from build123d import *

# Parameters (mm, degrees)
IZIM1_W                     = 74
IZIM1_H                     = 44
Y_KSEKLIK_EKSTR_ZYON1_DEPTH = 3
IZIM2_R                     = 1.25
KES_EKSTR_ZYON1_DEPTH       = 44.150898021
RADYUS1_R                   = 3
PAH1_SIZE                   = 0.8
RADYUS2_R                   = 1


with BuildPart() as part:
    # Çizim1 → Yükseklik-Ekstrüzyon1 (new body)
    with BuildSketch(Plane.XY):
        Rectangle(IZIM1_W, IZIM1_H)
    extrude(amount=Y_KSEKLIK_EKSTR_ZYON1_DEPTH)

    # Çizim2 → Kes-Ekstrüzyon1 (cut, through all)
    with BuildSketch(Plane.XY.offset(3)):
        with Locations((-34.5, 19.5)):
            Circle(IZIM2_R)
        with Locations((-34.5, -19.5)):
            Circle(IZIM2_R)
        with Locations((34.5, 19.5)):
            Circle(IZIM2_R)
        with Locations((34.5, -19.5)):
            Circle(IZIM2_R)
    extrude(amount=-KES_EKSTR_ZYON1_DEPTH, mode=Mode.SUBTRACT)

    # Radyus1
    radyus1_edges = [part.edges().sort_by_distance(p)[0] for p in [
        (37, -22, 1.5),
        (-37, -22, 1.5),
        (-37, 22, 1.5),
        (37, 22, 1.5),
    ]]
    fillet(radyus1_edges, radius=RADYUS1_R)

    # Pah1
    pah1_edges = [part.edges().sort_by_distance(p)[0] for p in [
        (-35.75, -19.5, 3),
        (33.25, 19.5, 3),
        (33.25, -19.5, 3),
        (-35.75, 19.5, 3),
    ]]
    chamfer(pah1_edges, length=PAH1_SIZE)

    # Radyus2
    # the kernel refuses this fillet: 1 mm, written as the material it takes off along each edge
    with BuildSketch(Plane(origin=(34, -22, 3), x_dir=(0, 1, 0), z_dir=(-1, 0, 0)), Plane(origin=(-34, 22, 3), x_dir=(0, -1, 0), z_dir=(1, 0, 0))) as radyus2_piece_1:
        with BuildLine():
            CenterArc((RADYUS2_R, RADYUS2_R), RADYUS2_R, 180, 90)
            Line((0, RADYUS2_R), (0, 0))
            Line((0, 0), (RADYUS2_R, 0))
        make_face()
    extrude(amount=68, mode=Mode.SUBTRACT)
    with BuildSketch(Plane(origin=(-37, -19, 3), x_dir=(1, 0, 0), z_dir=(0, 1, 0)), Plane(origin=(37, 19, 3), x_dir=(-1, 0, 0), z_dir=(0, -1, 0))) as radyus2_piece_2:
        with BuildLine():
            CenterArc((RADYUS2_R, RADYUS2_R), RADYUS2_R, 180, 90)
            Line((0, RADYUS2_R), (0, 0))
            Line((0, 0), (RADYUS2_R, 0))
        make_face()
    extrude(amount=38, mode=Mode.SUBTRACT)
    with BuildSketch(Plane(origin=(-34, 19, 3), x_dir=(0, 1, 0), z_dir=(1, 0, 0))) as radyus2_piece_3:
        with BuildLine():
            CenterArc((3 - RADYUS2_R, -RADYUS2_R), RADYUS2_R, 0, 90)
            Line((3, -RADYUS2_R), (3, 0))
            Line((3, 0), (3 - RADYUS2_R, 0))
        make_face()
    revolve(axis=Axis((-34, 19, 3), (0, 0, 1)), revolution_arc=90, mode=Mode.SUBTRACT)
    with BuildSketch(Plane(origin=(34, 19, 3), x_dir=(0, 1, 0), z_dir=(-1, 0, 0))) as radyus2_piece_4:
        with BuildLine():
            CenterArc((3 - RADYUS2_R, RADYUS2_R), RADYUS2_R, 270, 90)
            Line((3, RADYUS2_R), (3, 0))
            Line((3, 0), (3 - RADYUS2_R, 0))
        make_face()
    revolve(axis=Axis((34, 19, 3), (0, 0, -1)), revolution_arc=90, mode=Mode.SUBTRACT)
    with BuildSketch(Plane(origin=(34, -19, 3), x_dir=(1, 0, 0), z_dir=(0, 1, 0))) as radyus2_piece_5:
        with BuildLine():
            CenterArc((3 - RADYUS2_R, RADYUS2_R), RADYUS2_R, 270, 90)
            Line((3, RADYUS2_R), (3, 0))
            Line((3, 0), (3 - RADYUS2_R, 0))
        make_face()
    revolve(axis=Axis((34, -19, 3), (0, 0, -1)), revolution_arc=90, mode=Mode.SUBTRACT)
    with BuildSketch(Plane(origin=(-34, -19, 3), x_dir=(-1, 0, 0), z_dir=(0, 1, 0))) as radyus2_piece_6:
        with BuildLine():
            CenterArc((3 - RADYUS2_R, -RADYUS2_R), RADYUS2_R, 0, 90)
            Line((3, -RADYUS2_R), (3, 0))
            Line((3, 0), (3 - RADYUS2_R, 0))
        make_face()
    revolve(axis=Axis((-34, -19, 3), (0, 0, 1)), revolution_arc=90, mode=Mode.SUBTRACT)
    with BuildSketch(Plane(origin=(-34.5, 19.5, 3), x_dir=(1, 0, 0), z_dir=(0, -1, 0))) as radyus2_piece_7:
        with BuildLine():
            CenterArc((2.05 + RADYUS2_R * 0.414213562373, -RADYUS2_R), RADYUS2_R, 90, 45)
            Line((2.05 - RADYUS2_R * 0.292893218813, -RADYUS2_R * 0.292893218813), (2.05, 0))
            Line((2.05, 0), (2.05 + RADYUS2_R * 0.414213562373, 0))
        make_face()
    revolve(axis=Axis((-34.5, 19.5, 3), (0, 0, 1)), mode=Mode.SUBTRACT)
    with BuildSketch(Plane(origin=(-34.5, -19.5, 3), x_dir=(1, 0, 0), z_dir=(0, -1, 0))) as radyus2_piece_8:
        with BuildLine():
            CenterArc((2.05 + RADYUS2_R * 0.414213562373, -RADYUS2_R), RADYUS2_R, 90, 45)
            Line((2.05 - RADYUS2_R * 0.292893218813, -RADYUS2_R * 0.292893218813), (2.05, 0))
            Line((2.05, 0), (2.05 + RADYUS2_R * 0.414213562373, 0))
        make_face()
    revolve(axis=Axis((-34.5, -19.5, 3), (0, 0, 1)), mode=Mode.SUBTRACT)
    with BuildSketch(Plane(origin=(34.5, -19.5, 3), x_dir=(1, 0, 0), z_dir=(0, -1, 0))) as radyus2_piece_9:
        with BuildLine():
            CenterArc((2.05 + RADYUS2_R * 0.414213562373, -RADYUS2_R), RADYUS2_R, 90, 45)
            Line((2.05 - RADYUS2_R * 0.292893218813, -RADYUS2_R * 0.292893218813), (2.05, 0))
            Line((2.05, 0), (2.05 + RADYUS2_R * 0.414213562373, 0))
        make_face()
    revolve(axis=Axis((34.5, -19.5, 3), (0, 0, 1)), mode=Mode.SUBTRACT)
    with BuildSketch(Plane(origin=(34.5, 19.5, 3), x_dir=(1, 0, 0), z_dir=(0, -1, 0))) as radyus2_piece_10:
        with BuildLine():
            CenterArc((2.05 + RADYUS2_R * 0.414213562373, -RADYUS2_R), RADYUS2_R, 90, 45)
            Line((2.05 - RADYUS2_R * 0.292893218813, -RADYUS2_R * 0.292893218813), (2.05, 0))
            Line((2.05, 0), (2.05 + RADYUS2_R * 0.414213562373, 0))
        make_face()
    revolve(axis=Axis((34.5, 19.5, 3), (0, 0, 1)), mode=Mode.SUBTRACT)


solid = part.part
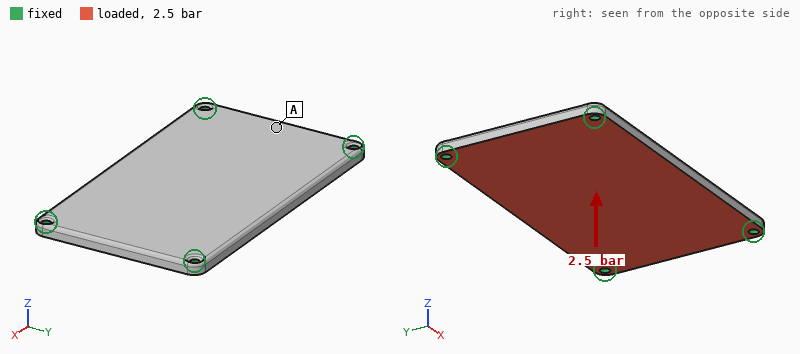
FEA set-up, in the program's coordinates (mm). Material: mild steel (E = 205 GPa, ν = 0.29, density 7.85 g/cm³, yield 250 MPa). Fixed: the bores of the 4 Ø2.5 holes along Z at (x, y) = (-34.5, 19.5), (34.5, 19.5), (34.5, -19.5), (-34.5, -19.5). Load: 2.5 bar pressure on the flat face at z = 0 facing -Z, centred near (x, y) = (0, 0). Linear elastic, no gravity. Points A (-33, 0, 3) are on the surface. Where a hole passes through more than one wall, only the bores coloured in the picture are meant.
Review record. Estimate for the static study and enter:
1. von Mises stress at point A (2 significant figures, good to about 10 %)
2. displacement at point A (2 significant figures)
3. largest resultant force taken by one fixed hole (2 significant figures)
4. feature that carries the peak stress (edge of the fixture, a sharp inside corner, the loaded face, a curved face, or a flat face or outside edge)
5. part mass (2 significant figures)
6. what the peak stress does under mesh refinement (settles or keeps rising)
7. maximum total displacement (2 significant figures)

21 MPa
9.9 µm
220 N
edge of the fixture
76 g
keeps rising
57 µm
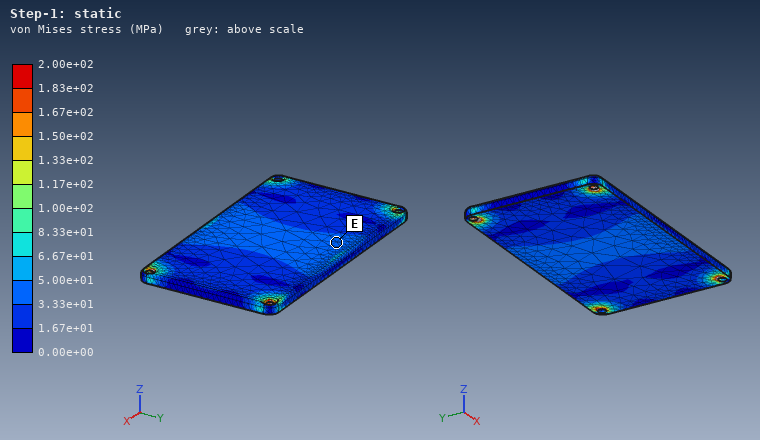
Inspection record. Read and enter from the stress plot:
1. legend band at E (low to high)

3.33e+01 to 5.00e+01 MPa
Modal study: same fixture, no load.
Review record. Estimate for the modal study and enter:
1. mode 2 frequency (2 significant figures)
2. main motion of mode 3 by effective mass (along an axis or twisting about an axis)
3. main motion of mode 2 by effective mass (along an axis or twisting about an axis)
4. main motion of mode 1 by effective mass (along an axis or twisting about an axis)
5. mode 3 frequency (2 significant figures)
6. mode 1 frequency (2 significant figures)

4500 Hz
twisting about Y
twisting about X
along Z
6600 Hz
2500 Hz
